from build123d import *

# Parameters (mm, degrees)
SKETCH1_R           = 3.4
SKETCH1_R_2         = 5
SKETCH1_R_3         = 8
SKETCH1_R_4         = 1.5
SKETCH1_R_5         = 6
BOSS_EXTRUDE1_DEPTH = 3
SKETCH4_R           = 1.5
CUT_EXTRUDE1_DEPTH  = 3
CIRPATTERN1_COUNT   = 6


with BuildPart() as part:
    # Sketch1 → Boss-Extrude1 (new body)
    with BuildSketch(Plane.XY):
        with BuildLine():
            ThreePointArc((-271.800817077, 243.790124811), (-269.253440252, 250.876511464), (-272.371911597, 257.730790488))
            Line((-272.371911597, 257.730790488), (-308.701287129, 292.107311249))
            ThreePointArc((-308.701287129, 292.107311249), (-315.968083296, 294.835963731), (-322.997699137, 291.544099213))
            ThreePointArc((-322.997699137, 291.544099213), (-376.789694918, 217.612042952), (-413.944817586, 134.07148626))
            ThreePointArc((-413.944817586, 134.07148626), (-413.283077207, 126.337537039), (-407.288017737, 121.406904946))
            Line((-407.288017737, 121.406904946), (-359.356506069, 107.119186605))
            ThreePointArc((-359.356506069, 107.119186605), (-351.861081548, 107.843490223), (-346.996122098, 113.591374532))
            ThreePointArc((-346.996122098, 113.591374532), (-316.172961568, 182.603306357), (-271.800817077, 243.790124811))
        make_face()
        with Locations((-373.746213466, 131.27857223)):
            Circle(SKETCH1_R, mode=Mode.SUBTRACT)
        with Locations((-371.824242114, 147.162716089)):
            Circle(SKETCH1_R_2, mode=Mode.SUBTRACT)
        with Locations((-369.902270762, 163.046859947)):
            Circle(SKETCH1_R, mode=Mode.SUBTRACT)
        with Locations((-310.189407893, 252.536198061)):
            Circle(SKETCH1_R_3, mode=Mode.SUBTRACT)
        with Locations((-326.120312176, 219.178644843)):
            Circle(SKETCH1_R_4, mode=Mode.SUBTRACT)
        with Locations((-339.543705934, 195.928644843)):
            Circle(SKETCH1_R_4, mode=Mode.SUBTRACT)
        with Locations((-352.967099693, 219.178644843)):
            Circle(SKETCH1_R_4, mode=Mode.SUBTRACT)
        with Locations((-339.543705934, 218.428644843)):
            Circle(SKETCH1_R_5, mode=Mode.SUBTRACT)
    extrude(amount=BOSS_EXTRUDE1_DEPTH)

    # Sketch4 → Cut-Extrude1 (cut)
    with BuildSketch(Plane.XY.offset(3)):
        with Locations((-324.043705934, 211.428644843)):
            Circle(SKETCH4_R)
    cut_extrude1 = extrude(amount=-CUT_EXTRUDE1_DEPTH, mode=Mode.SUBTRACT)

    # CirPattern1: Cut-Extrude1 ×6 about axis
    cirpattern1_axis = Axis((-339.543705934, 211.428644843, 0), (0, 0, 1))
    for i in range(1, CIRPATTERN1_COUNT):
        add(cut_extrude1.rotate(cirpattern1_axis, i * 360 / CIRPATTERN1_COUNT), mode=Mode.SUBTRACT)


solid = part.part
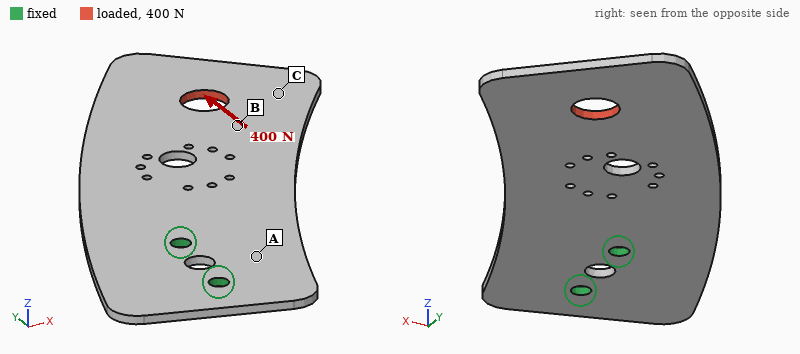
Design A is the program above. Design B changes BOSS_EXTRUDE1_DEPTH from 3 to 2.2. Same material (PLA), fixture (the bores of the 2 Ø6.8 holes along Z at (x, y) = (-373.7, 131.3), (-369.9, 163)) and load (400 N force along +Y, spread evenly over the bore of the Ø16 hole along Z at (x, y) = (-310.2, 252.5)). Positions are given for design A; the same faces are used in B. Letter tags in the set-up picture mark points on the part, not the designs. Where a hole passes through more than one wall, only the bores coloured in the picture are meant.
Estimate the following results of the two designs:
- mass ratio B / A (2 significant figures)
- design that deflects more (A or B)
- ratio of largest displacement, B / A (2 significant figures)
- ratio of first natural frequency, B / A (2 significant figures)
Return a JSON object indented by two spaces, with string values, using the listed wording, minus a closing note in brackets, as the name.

{
  "mass ratio B / A": "0.73",
  "design that deflects more": "B",
  "ratio of largest displacement, B / A": "1.4",
  "ratio of first natural frequency, B / A": "0.74"
}
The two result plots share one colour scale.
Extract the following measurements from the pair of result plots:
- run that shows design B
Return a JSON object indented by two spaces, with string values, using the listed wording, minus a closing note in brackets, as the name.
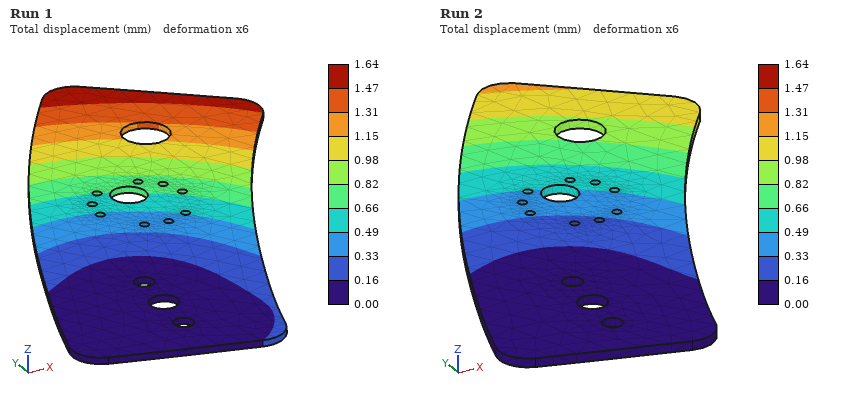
{
  "run that shows design B": "Run 1"
}
